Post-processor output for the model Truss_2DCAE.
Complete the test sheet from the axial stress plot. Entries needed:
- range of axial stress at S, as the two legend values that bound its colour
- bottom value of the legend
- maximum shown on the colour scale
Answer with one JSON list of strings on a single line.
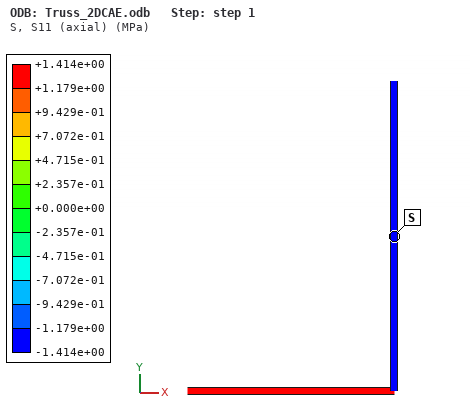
["-1.414e+00 to -1.179e+00 MPa", "-1.414e+00 MPa", "+1.414e+00 MPa"]
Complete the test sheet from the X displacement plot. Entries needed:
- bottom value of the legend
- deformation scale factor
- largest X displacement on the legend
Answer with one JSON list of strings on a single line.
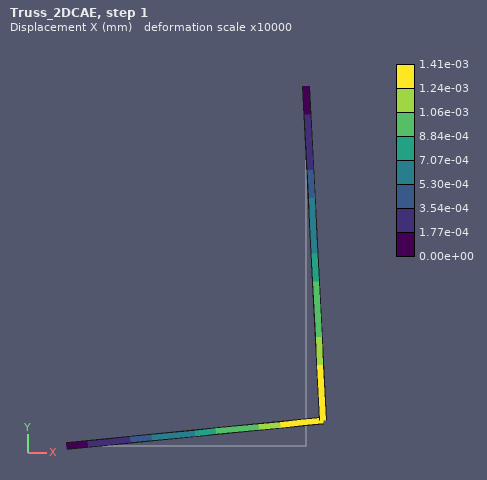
["0.00e+00 mm", "10000", "1.41e-03 mm"]
